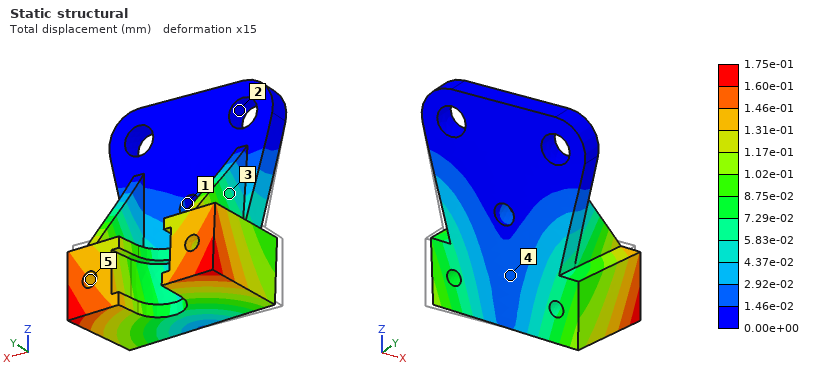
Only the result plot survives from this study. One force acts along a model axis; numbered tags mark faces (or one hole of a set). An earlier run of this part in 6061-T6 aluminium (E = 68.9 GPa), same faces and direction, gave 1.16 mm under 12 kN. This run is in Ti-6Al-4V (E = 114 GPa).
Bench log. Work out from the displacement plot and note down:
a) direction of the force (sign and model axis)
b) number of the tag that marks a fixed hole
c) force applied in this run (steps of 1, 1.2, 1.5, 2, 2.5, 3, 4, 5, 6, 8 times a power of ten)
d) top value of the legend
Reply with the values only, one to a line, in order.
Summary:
+X
2
3 kN
1.75e-01 mm
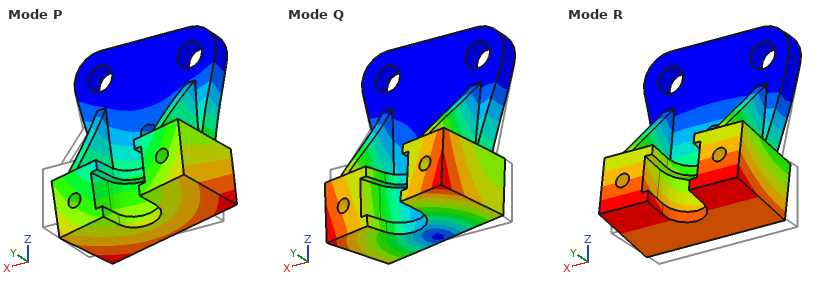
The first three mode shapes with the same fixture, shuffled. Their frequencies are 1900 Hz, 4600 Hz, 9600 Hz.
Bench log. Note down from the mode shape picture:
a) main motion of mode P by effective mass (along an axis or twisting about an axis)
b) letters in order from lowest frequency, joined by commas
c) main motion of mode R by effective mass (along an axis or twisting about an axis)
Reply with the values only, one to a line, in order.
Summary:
along X
R, Q, P
along Y
